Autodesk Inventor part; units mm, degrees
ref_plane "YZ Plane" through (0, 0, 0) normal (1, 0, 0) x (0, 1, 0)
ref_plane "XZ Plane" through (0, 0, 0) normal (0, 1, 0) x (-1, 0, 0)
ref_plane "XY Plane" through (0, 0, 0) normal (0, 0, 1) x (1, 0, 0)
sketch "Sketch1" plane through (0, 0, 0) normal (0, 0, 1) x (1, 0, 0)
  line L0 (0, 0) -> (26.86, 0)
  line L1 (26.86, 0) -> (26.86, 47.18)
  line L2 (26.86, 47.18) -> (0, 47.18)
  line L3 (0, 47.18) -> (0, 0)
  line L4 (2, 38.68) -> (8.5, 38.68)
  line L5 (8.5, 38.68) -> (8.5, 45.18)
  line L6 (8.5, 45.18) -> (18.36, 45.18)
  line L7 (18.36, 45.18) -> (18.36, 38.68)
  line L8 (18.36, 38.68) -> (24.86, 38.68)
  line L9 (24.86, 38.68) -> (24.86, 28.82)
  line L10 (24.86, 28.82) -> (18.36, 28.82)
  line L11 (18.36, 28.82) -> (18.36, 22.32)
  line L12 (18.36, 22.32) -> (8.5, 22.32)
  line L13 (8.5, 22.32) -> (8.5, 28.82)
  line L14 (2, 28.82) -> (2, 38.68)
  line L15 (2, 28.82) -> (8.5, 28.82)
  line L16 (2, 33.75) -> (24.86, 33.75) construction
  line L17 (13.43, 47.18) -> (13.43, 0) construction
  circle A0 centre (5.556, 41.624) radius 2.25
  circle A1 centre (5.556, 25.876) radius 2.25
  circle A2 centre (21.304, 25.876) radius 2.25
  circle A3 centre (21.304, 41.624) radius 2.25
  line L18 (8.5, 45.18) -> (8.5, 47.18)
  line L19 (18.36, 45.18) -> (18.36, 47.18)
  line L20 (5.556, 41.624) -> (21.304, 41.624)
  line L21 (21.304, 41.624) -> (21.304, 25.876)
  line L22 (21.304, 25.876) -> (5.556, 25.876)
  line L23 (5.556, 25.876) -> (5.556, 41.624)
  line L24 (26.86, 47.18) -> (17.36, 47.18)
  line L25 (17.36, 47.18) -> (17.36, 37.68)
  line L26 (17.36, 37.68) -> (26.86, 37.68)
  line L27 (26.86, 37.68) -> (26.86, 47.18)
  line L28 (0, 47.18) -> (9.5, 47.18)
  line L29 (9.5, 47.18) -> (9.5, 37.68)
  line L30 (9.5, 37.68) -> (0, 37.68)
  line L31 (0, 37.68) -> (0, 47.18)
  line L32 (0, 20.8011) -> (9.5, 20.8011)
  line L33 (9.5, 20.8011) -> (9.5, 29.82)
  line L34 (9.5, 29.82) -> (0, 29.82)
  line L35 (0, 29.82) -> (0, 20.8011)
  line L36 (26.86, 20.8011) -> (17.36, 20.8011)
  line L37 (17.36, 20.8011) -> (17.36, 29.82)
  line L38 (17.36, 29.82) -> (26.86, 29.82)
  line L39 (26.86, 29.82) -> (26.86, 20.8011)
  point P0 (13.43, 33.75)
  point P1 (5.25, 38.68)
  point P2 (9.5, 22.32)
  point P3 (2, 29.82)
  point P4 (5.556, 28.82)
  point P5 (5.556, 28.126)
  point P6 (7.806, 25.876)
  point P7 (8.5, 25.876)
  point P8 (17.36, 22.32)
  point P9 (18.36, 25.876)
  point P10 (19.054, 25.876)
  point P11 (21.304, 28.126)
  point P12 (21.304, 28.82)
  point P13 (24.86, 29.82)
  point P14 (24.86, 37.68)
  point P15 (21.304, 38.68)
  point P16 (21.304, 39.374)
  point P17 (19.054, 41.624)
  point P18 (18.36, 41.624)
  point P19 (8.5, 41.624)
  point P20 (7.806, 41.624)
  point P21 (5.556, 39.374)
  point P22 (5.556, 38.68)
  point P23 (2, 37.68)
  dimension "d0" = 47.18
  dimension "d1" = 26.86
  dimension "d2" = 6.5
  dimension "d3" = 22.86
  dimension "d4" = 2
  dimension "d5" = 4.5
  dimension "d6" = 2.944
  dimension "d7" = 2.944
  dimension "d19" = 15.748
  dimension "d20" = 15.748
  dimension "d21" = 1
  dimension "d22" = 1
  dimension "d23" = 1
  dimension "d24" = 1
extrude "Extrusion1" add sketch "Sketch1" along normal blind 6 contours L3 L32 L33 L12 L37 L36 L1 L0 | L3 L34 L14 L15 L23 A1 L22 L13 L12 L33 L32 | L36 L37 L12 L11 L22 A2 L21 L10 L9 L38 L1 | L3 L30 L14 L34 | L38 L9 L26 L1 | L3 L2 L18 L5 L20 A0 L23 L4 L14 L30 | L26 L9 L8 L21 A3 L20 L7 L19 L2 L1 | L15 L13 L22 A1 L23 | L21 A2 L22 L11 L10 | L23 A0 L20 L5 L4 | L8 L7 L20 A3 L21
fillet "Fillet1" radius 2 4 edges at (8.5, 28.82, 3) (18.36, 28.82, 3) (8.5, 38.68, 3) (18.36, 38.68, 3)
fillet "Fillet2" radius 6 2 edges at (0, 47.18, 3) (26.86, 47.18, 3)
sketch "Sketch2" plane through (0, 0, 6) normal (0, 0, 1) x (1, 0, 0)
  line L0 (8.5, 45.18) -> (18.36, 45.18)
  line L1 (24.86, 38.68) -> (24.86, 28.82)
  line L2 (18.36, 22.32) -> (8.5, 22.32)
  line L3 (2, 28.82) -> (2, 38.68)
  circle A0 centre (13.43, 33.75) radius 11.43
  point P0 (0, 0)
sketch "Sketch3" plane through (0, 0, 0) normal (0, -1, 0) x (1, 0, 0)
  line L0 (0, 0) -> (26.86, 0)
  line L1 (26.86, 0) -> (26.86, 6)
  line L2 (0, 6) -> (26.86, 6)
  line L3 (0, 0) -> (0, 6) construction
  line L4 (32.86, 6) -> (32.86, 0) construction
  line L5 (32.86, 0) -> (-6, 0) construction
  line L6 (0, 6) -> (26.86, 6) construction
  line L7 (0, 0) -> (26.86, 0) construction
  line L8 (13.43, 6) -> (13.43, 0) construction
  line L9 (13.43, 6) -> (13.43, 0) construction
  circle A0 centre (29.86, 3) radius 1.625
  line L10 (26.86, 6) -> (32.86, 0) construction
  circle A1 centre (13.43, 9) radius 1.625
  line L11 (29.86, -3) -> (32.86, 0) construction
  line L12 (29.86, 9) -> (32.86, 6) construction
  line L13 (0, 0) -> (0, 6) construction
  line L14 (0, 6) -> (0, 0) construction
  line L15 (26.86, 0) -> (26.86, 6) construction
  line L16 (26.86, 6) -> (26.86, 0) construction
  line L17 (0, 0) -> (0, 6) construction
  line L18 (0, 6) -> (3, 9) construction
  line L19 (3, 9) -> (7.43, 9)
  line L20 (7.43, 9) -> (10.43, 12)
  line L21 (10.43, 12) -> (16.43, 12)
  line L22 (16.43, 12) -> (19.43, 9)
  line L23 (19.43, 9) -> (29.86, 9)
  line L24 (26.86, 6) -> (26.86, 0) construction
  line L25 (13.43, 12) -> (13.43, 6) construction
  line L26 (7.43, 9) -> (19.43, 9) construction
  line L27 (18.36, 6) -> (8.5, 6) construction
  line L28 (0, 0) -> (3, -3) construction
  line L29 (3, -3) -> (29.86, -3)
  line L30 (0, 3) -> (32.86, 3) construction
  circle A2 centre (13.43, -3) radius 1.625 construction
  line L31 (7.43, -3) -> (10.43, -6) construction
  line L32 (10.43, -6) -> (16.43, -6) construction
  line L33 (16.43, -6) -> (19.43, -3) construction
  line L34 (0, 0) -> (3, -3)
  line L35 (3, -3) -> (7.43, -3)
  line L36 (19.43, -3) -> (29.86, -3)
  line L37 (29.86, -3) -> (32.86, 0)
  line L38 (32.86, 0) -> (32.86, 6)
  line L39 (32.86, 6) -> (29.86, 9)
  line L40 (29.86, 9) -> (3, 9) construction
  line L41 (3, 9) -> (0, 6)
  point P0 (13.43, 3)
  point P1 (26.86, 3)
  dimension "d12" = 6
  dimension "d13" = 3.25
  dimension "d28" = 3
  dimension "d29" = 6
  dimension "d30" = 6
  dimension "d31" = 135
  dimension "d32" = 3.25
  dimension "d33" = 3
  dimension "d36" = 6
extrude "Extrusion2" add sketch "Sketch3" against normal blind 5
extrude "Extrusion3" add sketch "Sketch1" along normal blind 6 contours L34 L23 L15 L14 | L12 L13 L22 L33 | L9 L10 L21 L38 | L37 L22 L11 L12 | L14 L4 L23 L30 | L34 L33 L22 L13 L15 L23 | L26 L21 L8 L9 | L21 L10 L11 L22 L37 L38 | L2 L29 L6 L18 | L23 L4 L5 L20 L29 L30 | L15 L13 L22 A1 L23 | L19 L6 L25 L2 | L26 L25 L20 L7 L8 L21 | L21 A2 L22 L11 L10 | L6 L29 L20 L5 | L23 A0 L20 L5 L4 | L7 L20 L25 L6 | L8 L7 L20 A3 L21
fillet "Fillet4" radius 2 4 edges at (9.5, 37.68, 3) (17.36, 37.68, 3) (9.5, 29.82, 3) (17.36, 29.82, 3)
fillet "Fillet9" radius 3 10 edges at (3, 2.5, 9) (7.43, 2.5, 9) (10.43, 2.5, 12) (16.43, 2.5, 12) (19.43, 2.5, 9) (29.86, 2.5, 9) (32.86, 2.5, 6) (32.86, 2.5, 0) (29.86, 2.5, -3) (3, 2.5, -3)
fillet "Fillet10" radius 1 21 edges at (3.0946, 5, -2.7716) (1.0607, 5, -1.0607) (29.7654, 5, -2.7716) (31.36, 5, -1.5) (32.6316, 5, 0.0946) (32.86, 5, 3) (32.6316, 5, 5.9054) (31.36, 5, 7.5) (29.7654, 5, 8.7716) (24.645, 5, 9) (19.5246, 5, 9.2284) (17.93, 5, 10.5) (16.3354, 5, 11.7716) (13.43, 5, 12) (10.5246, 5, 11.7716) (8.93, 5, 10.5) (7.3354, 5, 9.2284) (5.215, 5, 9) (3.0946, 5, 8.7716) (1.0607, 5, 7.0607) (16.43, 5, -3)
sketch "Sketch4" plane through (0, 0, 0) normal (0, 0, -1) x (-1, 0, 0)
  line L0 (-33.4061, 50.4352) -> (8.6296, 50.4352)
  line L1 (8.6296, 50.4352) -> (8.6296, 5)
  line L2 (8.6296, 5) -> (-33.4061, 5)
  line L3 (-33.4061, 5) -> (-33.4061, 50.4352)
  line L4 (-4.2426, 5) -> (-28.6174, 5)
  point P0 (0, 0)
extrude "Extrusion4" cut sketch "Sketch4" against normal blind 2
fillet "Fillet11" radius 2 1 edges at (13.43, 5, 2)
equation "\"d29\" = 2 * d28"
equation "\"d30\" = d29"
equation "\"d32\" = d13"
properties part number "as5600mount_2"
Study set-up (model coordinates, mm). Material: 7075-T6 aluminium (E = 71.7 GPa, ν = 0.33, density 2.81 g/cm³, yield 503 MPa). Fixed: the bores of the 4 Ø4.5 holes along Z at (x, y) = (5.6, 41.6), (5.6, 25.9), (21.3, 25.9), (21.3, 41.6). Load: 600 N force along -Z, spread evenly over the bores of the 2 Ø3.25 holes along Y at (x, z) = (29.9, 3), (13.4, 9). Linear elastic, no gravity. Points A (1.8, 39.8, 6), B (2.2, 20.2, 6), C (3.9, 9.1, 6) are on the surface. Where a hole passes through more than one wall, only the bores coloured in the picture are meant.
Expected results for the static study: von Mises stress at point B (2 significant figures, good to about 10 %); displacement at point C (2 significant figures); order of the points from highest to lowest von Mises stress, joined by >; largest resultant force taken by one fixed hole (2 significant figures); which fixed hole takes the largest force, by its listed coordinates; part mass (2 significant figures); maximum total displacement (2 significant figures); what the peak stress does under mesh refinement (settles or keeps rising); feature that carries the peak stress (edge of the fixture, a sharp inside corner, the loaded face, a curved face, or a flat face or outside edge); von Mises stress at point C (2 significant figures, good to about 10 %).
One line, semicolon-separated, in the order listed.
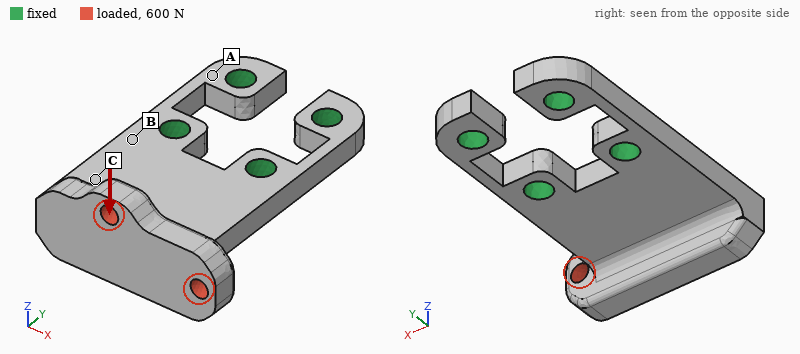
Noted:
140 MPa; 0.12 mm; B > C > A; 560 N; (21.3, 25.9); 14 g; 0.38 mm; keeps rising; edge of the fixture; 72 MPa
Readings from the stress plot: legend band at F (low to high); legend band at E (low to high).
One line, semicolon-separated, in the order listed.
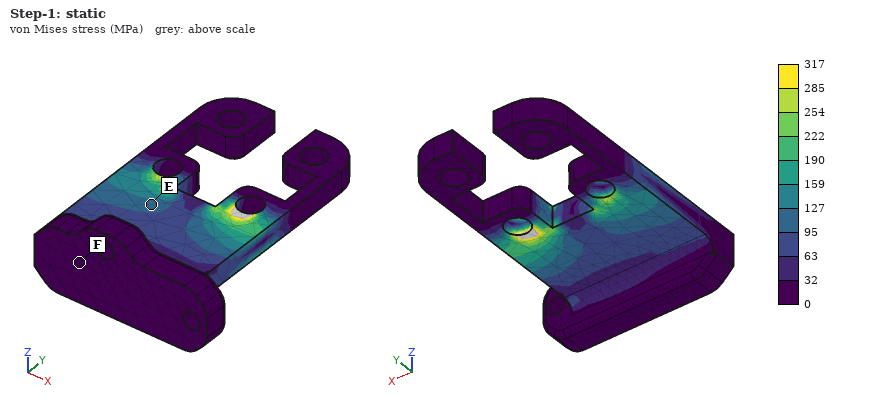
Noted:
0 to 32 MPa; 95 to 127 MPa
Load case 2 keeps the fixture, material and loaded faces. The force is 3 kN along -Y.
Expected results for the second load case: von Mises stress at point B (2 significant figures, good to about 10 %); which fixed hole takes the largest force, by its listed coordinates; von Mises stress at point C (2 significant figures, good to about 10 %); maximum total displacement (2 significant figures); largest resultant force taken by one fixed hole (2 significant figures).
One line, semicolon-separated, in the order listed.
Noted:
85 MPa; (21.3, 25.9); 77 MPa; 0.23 mm; 2.8 kN
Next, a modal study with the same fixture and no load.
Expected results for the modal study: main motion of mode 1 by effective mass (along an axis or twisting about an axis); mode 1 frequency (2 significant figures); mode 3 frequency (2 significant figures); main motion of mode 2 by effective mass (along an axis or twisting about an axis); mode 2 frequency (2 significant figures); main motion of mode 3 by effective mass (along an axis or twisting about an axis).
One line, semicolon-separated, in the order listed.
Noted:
along Z; 3000 Hz; 13 kHz; twisting about Y; 7300 Hz; along X
